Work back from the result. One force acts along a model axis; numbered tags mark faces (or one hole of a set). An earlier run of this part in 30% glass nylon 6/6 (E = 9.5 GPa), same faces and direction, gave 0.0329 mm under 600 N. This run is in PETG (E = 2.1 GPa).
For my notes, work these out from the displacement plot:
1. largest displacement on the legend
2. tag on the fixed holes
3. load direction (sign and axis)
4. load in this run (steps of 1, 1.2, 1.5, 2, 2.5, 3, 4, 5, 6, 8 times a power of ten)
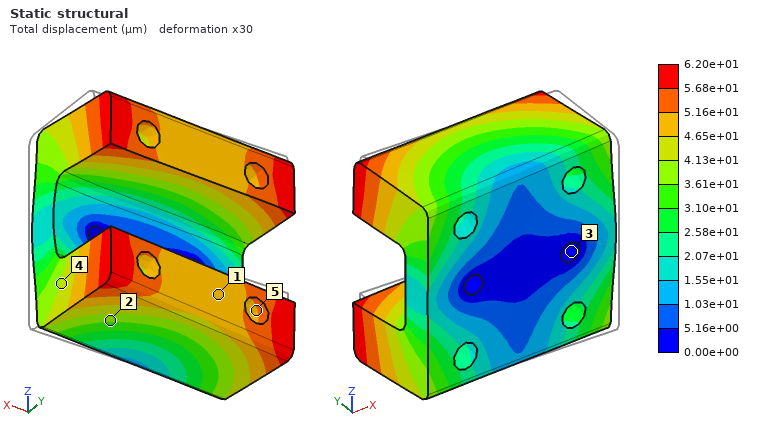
6.20e+01 µm
3
-X
250 N
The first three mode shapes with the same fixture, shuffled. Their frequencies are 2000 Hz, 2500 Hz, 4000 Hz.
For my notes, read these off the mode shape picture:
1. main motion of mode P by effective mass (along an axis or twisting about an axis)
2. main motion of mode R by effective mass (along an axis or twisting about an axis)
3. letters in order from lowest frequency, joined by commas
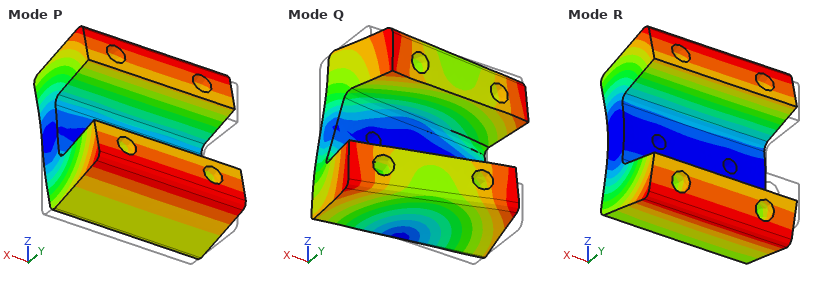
along Z
along Y
P, R, Q
